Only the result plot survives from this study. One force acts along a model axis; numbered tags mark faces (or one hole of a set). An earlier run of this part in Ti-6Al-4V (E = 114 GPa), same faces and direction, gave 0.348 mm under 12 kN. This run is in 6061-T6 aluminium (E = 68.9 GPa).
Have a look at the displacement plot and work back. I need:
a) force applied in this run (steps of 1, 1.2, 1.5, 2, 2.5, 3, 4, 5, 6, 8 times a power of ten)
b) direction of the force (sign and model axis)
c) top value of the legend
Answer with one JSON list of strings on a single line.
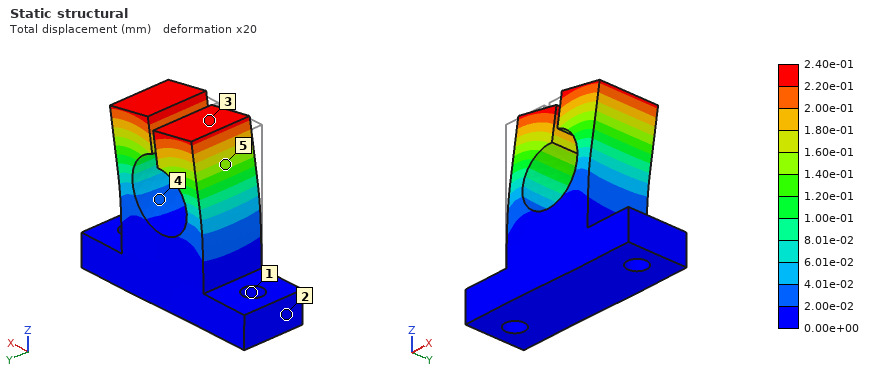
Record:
["5 kN", "+X", "2.40e-01 mm"]
